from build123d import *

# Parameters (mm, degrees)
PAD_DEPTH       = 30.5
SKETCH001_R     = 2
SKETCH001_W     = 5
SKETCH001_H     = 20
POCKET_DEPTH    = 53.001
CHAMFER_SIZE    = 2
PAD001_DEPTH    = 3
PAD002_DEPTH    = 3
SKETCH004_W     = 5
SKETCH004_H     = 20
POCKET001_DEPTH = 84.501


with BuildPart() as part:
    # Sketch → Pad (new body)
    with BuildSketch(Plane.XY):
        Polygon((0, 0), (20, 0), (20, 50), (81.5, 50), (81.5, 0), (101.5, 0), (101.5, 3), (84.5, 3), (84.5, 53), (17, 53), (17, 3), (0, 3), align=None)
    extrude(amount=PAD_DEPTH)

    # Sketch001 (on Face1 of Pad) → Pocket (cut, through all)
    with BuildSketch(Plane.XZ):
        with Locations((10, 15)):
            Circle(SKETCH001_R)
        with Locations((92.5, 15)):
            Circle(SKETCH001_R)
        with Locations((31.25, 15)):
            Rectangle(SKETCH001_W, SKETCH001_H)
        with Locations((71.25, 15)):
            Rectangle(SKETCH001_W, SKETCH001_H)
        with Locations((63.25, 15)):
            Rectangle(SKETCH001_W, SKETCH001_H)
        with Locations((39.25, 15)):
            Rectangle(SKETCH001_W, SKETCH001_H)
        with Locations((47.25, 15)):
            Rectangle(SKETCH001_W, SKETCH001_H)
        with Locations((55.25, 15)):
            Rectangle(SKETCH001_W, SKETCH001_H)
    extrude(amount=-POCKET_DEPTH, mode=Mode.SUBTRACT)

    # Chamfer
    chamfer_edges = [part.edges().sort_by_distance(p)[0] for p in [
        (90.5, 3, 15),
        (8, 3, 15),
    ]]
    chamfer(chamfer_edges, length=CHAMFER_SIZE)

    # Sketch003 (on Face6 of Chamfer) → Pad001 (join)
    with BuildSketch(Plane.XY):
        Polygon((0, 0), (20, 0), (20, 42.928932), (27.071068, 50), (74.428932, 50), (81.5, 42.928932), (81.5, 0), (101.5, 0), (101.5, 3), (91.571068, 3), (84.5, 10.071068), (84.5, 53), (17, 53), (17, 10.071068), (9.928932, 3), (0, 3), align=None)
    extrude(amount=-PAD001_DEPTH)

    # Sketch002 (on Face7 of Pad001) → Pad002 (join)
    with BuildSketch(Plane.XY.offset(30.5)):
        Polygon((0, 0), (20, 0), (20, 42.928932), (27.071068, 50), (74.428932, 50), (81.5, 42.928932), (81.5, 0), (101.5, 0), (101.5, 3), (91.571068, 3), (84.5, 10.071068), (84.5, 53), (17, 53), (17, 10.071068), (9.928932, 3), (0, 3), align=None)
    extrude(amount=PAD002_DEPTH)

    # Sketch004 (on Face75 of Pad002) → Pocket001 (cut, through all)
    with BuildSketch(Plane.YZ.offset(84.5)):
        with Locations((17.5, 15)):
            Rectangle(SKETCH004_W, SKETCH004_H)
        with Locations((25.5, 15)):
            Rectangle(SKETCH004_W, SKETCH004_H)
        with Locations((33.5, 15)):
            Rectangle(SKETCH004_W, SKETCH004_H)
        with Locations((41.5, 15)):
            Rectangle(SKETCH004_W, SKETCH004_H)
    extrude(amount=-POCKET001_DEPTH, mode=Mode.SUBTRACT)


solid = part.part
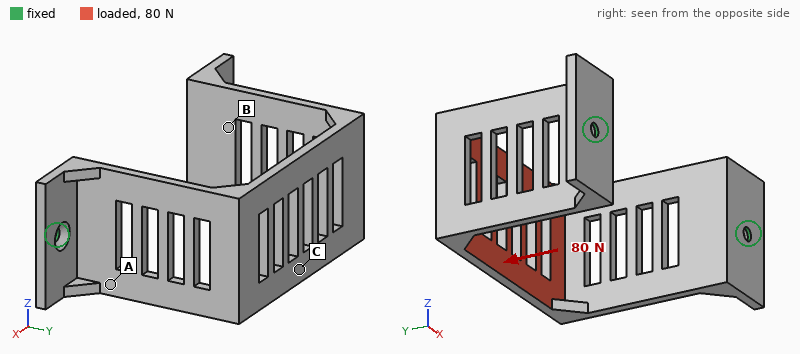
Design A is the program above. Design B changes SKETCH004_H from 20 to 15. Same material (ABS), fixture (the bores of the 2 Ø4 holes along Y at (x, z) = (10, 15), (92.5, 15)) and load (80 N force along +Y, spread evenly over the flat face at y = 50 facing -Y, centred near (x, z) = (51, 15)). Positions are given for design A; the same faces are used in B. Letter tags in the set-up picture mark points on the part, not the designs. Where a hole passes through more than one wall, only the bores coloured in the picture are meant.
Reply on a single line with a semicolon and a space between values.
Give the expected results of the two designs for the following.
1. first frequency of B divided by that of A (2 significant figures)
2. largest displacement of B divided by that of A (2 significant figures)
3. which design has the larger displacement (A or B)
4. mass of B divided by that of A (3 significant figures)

0.99; 0.91; A; 1.03
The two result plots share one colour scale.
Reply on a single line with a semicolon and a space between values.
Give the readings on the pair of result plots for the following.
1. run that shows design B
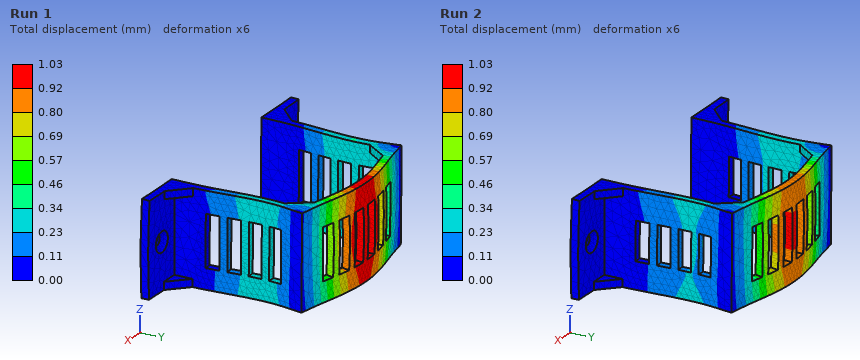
Run 2
